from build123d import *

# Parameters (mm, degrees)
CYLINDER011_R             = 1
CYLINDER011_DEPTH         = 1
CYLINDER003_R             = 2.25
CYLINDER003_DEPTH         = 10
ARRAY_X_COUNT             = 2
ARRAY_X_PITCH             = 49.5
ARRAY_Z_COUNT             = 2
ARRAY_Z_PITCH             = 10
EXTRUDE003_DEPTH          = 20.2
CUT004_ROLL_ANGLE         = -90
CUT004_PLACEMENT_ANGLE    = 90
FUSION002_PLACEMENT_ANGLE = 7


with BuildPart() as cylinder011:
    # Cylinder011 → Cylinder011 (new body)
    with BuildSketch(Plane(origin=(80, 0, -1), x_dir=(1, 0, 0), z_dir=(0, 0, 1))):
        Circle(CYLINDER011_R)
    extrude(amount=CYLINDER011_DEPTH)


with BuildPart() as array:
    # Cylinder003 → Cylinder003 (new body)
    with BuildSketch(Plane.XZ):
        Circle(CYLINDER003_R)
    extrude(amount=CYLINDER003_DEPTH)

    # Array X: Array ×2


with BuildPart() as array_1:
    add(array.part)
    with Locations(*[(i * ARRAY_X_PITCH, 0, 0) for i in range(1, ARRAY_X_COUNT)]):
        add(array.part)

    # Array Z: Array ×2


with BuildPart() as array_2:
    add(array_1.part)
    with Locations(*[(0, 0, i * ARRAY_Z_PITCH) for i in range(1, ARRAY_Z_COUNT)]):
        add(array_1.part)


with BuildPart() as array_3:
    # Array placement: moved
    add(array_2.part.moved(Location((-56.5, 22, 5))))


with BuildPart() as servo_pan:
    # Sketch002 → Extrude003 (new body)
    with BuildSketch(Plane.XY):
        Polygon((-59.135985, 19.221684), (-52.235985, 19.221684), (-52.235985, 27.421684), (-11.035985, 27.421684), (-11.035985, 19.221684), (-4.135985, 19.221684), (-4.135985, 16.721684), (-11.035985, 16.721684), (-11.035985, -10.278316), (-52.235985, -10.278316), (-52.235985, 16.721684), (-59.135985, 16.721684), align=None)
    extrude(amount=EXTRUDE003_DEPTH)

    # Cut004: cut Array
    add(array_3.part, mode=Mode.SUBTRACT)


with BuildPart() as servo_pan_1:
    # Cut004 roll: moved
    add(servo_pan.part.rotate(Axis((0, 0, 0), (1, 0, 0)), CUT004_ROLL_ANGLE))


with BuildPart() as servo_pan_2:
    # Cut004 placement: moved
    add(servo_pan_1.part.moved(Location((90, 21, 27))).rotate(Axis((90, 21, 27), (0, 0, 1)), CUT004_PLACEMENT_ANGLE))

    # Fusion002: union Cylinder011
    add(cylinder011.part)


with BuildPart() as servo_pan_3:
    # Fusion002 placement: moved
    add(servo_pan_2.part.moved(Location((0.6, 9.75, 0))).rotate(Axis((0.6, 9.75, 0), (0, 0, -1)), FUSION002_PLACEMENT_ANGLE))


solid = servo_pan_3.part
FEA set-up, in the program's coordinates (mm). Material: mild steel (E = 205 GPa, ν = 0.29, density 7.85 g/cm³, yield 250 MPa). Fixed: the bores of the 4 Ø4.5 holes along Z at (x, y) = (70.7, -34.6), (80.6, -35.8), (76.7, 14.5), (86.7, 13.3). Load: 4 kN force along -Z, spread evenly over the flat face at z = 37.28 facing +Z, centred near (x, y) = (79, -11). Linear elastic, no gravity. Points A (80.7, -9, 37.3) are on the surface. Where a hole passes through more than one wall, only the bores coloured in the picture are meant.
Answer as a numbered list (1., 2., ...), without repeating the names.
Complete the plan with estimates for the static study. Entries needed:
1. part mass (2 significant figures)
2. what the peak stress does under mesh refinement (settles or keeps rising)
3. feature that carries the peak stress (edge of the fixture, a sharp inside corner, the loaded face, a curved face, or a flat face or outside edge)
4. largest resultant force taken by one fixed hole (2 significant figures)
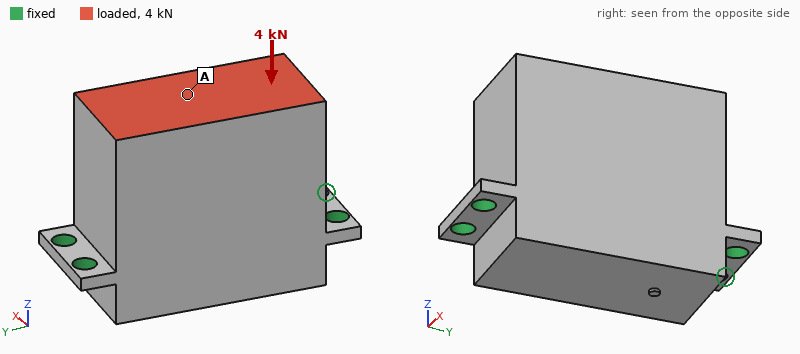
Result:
1. 250 g
2. keeps rising
3. edge of the fixture
4. 1.0 kN
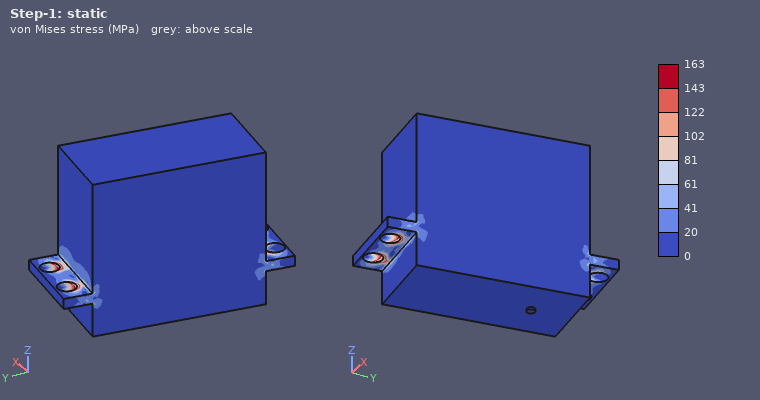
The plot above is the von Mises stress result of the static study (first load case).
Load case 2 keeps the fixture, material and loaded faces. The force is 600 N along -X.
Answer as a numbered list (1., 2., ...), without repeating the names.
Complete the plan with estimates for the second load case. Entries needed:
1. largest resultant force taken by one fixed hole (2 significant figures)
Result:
1. 750 N
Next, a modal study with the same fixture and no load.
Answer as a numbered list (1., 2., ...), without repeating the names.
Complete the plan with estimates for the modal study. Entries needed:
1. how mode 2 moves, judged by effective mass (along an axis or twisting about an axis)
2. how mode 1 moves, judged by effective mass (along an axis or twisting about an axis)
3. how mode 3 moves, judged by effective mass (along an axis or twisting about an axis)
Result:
1. along Z
2. along X
3. along Y
